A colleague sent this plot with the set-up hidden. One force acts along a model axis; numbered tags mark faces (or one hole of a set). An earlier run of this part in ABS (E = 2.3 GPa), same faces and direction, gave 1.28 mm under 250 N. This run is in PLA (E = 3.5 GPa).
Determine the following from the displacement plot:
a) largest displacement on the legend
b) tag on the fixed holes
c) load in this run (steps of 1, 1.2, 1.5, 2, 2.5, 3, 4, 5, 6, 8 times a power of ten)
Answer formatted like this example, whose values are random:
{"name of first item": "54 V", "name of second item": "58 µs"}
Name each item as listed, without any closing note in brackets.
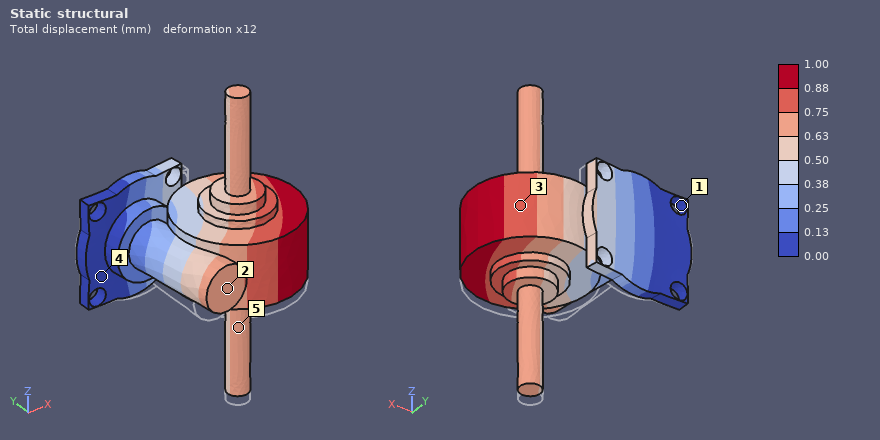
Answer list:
{"largest displacement on the legend": "1.00 mm", "tag on the fixed holes": "1", "load in this run": "300 N"}
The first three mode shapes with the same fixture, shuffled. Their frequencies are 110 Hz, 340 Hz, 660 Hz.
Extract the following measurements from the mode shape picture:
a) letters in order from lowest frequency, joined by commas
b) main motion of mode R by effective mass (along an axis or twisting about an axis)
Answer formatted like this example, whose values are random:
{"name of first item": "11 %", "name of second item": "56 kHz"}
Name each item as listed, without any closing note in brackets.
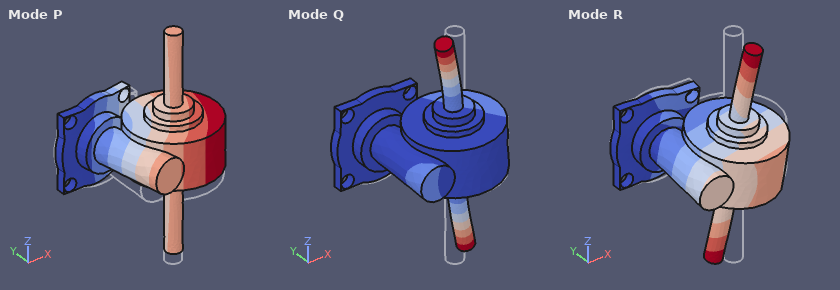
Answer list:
{"letters in order from lowest frequency, joined by commas": "P, R, Q", "main motion of mode R by effective mass": "along Z"}
